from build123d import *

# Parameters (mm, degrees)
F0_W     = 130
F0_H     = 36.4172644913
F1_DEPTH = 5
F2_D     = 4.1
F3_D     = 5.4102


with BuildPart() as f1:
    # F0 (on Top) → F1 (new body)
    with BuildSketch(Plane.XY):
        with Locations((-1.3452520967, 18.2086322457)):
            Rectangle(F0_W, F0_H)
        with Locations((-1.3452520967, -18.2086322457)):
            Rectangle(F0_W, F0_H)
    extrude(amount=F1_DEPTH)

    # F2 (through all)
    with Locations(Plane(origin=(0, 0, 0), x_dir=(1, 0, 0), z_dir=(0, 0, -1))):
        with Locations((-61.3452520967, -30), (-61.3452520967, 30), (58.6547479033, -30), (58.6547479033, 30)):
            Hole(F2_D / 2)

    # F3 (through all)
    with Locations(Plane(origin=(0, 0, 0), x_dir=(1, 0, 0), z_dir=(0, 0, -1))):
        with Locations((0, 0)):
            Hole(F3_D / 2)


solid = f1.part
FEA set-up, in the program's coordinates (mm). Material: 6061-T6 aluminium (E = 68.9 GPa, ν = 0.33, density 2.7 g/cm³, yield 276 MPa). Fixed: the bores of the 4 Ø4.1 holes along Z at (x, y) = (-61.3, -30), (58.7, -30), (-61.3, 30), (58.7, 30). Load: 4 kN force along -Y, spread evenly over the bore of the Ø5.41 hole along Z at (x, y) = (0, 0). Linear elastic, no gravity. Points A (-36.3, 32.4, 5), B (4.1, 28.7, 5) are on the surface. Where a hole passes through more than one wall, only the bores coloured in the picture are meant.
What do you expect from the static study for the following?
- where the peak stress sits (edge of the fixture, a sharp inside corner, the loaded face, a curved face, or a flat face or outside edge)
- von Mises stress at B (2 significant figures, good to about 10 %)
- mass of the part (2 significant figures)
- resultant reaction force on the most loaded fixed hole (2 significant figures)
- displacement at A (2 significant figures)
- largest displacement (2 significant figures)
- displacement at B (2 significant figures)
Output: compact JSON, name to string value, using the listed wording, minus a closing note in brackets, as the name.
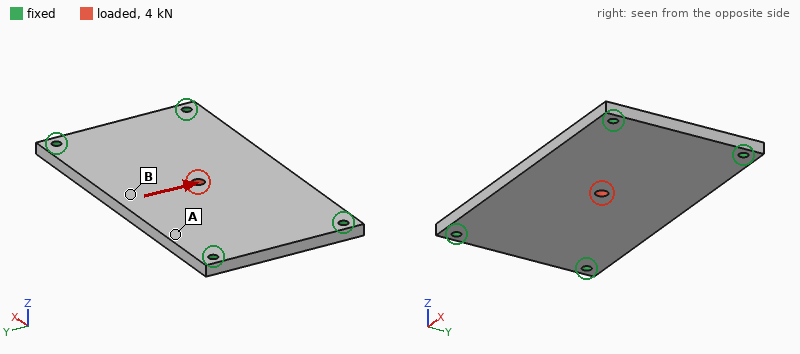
{"where the peak stress sits": "the loaded face", "von Mises stress at B": "10.0 MPa", "mass of the part": "130 g", "resultant reaction force on the most loaded fixed hole": "1.4 kN", "displacement at A": "9.8 µm", "largest displacement": "24 µm", "displacement at B": "17 µm"}
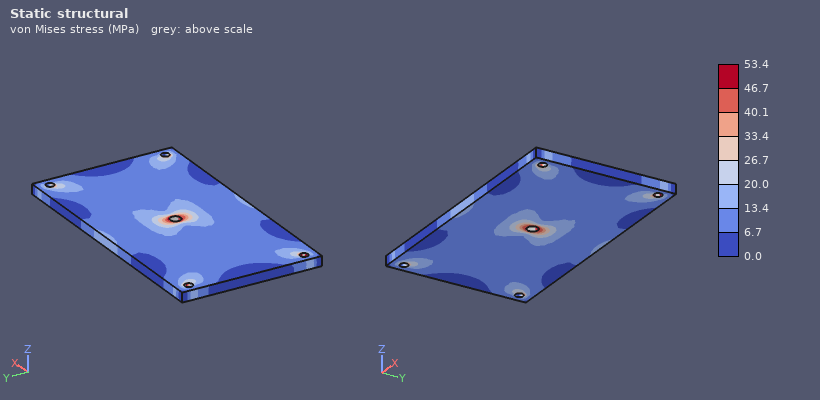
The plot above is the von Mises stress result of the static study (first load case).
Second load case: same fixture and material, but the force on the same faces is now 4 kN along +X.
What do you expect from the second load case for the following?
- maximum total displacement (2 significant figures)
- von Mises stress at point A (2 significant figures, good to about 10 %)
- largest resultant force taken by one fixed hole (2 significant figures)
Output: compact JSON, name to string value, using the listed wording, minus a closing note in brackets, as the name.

{"maximum total displacement": "13 µm", "von Mises stress at point A": "6.4 MPa", "largest resultant force taken by one fixed hole": "1.1 kN"}
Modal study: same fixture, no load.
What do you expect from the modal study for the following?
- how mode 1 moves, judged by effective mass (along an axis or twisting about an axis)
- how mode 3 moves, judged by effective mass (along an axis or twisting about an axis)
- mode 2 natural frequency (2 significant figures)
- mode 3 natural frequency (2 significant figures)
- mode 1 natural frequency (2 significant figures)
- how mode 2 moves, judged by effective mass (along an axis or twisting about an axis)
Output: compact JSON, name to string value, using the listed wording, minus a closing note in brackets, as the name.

{"how mode 1 moves, judged by effective mass": "along Z", "how mode 3 moves, judged by effective mass": "twisting about Y", "mode 2 natural frequency": "2600 Hz", "mode 3 natural frequency": "4100 Hz", "mode 1 natural frequency": "1500 Hz", "how mode 2 moves, judged by effective mass": "twisting about X"}
